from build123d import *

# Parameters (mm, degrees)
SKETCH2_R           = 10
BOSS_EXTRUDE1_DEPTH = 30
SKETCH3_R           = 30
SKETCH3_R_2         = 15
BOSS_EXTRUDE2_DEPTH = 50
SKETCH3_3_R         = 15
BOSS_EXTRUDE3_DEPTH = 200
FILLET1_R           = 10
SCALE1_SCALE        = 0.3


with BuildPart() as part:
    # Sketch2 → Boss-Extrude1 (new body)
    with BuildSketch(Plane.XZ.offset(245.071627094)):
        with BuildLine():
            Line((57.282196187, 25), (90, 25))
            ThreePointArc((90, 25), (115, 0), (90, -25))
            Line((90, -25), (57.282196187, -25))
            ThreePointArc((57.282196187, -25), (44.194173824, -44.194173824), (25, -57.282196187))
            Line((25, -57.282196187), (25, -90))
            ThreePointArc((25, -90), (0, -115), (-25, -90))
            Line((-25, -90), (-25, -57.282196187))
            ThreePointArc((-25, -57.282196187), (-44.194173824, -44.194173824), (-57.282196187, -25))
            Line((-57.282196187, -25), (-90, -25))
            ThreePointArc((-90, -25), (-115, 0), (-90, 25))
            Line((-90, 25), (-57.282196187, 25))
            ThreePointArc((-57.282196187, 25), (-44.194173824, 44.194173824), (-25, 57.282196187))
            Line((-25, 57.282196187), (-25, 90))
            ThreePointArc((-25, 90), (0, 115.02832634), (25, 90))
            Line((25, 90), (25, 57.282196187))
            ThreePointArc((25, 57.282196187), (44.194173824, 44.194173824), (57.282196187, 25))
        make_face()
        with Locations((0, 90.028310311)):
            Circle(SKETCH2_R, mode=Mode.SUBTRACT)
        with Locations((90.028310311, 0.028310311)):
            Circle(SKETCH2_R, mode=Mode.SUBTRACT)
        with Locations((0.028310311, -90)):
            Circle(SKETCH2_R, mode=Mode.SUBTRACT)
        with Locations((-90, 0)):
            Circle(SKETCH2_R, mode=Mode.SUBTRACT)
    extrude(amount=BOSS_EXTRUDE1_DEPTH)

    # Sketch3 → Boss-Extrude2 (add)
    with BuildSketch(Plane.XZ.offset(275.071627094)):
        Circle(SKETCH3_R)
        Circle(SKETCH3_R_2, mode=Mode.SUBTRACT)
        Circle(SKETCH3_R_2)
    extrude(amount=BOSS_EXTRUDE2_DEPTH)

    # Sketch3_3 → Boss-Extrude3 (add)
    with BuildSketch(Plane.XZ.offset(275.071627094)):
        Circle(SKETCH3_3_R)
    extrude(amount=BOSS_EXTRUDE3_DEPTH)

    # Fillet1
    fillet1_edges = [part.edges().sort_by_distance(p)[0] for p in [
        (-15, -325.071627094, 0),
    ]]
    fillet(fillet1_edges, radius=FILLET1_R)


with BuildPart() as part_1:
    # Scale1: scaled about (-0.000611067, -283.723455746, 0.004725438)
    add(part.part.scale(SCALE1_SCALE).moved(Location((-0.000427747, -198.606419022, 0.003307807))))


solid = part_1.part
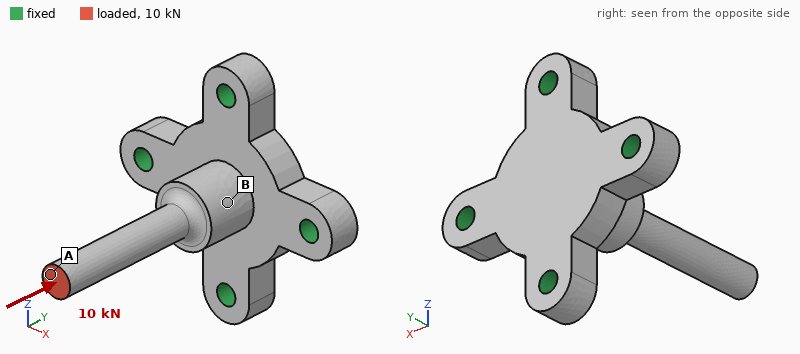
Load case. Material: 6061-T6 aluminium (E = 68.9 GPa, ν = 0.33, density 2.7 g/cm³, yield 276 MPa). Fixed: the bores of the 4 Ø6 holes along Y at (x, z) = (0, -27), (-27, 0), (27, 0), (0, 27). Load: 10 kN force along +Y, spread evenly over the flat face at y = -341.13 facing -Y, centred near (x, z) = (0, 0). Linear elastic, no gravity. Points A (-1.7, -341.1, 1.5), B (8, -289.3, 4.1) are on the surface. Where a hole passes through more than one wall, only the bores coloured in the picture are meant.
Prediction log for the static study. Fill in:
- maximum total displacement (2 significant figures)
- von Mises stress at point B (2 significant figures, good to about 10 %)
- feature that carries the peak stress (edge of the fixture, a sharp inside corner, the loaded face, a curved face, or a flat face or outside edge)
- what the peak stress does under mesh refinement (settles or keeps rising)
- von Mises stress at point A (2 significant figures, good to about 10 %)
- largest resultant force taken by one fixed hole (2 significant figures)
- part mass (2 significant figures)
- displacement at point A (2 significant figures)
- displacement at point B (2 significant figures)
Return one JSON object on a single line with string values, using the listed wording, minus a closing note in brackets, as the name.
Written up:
{"maximum total displacement": "0.15 mm", "von Mises stress at point B": "31 MPa", "feature that carries the peak stress": "edge of the fixture", "what the peak stress does under mesh refinement": "keeps rising", "von Mises stress at point A": "160 MPa", "largest resultant force taken by one fixed hole": "2.5 kN", "part mass": "64 g", "displacement at point A": "0.15 mm", "displacement at point B": "0.040 mm"}
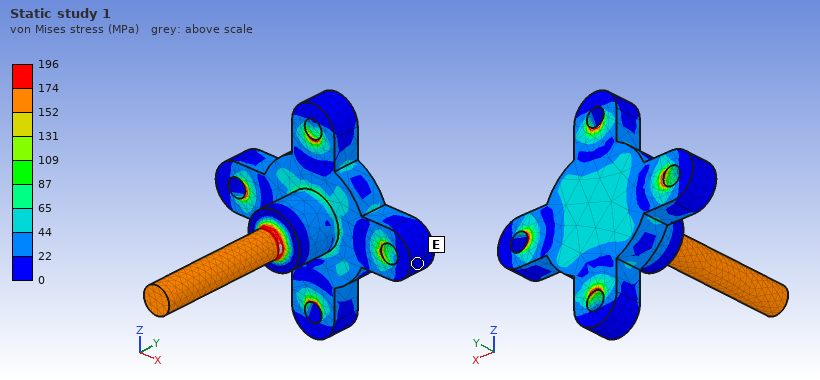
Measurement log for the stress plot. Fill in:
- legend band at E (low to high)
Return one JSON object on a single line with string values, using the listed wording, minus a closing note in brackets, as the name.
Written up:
{"legend band at E": "0 to 22 MPa"}
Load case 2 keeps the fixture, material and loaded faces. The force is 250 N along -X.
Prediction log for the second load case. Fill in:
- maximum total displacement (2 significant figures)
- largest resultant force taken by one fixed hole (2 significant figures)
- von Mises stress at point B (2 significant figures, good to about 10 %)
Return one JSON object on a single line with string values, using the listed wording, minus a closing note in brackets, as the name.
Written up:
{"maximum total displacement": "0.41 mm", "largest resultant force taken by one fixed hole": "380 N", "von Mises stress at point B": "19 MPa"}
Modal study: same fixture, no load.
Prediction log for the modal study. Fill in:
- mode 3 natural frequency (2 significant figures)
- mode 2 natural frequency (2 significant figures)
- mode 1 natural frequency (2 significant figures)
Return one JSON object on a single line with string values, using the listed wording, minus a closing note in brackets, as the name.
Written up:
{"mode 3 natural frequency": "12 kHz", "mode 2 natural frequency": "2800 Hz", "mode 1 natural frequency": "2800 Hz"}
